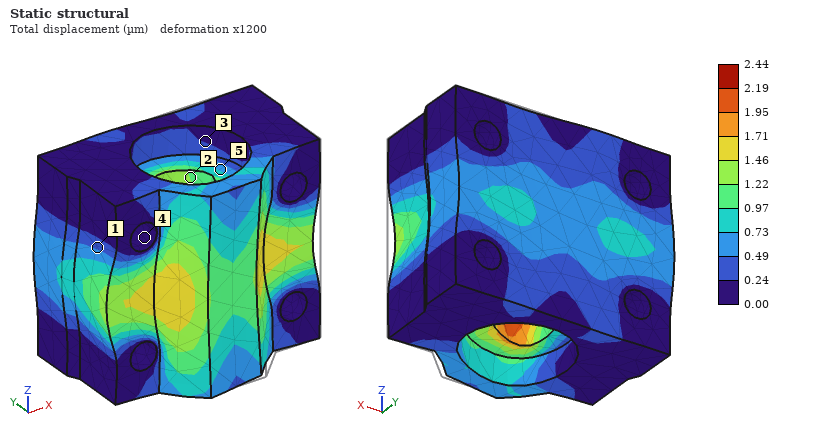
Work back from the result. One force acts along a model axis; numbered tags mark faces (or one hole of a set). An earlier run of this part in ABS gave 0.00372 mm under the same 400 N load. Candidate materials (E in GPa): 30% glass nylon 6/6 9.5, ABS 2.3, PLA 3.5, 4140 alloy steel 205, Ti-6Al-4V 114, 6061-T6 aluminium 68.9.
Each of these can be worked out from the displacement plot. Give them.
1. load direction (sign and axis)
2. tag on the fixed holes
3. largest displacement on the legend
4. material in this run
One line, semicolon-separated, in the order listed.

-X; 4; 2.44 µm; PLA
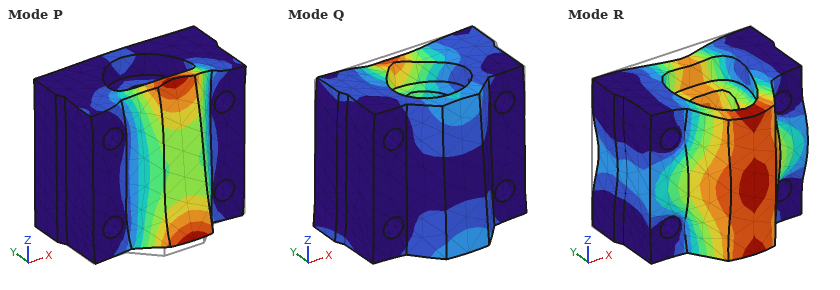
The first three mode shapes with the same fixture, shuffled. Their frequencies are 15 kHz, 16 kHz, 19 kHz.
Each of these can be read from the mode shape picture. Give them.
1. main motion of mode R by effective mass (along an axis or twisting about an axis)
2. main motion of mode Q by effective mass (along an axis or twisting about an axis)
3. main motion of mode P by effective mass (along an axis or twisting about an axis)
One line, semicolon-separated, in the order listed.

along Y; along Z; along Z
